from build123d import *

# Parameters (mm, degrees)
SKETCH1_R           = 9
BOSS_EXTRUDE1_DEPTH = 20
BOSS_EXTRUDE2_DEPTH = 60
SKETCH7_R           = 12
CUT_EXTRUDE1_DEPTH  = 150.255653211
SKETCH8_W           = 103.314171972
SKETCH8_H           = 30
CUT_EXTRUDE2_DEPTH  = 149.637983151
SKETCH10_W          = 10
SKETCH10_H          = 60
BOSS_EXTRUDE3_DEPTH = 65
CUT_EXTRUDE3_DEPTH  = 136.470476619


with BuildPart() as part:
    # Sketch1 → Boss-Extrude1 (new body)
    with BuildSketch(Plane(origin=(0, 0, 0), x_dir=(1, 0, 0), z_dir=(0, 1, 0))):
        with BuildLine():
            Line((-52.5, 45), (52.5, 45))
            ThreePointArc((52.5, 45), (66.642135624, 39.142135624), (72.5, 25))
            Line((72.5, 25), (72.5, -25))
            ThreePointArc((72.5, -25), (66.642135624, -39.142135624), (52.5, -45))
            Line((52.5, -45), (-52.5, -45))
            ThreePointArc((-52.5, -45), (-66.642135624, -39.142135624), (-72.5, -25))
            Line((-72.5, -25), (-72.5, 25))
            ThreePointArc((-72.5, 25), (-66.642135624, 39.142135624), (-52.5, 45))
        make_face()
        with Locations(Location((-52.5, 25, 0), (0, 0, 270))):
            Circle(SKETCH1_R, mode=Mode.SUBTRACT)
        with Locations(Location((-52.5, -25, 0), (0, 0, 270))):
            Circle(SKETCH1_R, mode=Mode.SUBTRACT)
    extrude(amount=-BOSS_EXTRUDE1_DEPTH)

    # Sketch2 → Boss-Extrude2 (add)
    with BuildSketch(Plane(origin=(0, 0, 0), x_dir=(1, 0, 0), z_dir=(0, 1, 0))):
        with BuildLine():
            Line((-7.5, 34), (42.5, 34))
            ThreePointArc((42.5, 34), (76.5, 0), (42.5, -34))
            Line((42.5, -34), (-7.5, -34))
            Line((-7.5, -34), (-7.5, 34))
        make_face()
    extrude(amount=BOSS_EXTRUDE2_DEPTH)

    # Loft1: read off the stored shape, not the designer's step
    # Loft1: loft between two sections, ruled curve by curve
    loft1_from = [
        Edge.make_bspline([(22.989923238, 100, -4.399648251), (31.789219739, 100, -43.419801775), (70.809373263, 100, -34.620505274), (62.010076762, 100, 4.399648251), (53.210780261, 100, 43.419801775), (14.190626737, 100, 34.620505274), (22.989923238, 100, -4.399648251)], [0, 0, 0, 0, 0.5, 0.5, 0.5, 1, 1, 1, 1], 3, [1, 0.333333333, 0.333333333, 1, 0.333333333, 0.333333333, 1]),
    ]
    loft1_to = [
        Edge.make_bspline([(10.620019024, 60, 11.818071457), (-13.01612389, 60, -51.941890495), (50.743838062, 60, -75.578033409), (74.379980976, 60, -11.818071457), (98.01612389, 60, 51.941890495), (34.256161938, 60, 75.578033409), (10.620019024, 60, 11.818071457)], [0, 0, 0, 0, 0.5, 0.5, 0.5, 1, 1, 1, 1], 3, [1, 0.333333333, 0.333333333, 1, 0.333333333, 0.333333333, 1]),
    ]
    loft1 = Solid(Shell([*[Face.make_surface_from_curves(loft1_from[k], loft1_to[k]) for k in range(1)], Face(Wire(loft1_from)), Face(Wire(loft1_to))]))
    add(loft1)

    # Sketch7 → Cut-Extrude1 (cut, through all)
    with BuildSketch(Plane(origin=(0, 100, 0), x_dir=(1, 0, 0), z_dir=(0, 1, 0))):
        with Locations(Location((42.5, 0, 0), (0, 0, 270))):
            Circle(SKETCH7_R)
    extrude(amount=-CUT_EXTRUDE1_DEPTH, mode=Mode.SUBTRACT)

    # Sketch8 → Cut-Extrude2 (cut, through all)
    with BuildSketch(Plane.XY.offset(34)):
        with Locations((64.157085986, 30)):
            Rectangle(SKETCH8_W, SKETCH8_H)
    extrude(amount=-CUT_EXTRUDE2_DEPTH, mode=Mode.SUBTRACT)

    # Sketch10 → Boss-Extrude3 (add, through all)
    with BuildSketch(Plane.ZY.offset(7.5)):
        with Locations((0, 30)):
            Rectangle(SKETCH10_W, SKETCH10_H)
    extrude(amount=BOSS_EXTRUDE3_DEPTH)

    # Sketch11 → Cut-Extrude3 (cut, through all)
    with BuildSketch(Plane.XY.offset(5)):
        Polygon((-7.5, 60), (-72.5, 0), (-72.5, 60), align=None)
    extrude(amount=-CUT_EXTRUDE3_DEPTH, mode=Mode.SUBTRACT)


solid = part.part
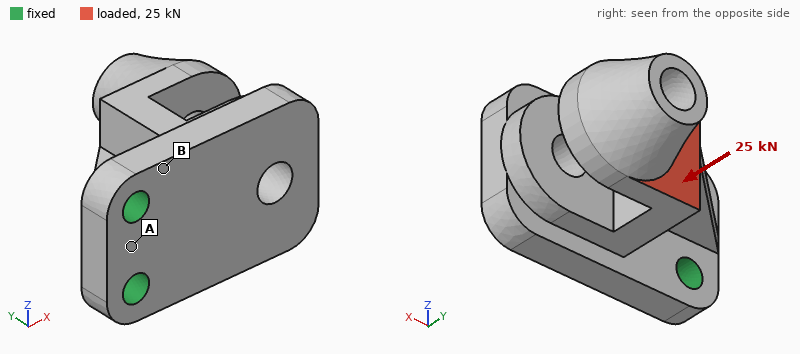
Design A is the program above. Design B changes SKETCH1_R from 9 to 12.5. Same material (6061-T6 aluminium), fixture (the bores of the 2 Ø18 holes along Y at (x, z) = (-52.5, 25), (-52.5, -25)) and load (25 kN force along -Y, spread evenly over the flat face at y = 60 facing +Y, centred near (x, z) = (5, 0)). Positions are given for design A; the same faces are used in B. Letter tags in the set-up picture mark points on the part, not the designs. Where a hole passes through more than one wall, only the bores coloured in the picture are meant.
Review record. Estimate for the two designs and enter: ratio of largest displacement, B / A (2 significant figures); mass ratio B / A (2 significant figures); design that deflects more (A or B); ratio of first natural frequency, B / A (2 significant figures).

0.79
0.98
A
1.1
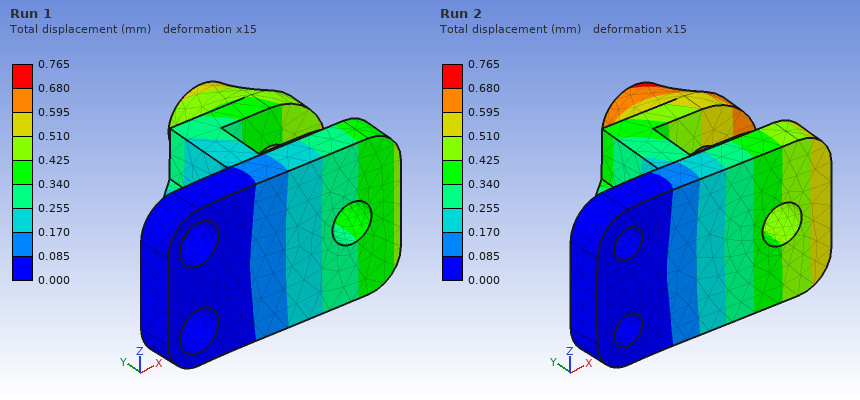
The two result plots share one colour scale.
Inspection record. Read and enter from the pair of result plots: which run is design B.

Run 1
